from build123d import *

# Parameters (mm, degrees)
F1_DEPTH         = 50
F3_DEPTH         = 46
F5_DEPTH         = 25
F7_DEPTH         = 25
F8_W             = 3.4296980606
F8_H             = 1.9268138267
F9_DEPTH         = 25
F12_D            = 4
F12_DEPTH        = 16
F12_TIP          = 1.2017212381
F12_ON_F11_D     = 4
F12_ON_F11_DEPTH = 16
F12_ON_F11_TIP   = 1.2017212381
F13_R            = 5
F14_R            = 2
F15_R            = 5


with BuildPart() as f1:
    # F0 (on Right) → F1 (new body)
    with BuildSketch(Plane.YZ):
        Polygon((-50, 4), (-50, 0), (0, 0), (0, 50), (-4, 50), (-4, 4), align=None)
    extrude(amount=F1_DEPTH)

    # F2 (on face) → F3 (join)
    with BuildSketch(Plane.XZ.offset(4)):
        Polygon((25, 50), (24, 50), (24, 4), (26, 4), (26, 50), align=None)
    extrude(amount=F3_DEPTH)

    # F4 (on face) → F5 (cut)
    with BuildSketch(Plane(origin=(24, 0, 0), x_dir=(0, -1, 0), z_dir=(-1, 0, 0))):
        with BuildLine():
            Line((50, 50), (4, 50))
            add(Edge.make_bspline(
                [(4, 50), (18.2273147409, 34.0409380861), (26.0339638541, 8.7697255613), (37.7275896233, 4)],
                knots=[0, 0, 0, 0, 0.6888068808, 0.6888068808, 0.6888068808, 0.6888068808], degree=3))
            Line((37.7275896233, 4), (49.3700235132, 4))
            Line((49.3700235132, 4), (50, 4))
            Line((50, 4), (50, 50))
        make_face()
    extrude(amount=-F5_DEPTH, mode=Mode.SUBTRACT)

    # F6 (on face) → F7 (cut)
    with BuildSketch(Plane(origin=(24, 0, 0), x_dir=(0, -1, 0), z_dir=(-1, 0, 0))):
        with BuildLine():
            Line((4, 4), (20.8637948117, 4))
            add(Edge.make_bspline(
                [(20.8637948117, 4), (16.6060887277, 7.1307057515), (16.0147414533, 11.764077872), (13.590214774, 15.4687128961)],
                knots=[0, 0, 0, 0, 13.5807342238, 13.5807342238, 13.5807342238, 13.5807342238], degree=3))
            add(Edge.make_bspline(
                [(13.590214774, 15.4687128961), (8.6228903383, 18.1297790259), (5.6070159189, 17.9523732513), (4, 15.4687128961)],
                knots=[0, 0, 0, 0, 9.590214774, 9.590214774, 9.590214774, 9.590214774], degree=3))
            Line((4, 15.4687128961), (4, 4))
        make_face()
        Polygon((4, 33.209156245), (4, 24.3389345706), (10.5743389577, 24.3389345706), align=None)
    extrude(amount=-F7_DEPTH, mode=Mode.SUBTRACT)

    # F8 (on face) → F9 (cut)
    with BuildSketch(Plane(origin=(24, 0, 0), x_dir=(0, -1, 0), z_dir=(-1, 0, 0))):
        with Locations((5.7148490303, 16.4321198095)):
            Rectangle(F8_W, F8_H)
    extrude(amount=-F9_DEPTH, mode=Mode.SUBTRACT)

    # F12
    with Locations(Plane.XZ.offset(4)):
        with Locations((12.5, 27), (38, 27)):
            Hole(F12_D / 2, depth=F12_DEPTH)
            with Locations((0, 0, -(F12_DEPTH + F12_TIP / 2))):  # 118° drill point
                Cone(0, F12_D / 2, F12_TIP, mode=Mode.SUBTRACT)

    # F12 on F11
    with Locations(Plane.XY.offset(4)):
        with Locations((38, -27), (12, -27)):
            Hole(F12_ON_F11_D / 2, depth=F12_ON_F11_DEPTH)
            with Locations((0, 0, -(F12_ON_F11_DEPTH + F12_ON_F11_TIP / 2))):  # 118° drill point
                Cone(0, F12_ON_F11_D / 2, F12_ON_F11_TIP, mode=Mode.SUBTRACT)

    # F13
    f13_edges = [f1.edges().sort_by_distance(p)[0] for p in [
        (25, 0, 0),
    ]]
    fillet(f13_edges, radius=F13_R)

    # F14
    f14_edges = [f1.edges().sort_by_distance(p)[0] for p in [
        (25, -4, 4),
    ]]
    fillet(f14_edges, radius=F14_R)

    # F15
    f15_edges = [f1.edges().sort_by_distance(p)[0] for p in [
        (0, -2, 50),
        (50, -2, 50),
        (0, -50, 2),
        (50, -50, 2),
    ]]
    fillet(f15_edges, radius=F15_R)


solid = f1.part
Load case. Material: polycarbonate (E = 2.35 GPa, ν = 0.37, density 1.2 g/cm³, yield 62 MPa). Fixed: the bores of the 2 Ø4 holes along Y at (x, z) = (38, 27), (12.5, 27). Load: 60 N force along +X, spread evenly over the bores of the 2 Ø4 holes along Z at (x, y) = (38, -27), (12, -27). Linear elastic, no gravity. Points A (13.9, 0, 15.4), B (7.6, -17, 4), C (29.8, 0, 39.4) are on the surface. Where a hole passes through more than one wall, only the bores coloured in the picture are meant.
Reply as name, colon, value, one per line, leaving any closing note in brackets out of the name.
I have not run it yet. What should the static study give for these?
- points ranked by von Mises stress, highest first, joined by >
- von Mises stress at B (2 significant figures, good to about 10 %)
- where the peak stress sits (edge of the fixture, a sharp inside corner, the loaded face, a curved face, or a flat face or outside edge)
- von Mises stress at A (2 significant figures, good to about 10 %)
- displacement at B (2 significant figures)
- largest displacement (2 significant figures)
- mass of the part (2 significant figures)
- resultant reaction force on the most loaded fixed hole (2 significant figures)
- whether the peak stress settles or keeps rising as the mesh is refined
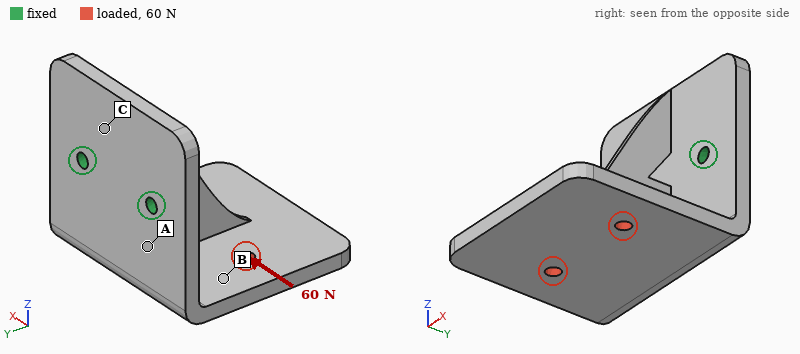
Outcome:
points ranked by von Mises stress, highest first, joined by >: A > B > C
von Mises stress at B: 2.3 MPa
where the peak stress sits: edge of the fixture
von Mises stress at A: 4.4 MPa
displacement at B: 0.42 mm
largest displacement: 0.95 mm
mass of the part: 24 g
resultant reaction force on the most loaded fixed hole: 78 N
whether the peak stress settles or keeps rising as the mesh is refined: keeps rising
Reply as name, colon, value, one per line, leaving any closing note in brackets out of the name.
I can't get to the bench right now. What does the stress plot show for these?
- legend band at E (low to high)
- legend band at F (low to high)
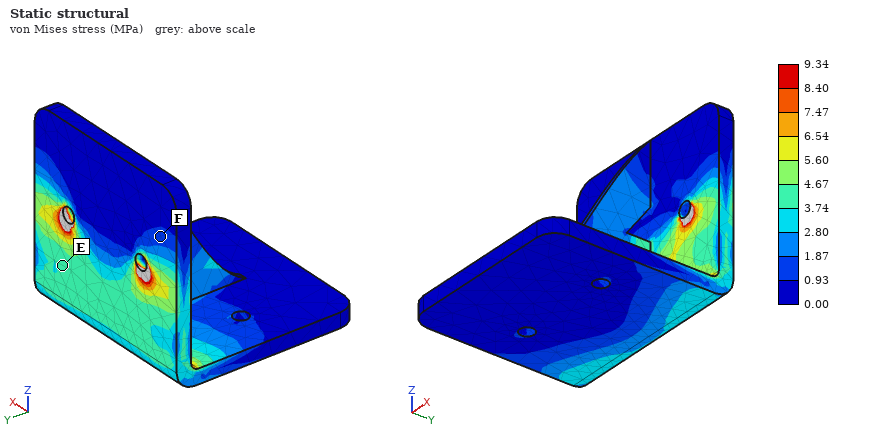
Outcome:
legend band at E: 3.74 to 4.67 MPa
legend band at F: 0.93 to 1.87 MPa
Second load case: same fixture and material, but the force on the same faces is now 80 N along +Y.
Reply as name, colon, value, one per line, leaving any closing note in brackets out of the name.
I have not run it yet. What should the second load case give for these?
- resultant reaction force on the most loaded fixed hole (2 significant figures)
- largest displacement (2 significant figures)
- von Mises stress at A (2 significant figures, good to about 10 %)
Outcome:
resultant reaction force on the most loaded fixed hole: 42 N
largest displacement: 0.90 mm
von Mises stress at A: 3.4 MPa
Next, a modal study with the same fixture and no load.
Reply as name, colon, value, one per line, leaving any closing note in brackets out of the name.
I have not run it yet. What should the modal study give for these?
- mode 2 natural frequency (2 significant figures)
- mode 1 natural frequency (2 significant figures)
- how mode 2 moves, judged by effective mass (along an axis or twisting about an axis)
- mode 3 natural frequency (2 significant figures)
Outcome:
mode 2 natural frequency: 420 Hz
mode 1 natural frequency: 410 Hz
how mode 2 moves, judged by effective mass: along X
mode 3 natural frequency: 880 Hz
